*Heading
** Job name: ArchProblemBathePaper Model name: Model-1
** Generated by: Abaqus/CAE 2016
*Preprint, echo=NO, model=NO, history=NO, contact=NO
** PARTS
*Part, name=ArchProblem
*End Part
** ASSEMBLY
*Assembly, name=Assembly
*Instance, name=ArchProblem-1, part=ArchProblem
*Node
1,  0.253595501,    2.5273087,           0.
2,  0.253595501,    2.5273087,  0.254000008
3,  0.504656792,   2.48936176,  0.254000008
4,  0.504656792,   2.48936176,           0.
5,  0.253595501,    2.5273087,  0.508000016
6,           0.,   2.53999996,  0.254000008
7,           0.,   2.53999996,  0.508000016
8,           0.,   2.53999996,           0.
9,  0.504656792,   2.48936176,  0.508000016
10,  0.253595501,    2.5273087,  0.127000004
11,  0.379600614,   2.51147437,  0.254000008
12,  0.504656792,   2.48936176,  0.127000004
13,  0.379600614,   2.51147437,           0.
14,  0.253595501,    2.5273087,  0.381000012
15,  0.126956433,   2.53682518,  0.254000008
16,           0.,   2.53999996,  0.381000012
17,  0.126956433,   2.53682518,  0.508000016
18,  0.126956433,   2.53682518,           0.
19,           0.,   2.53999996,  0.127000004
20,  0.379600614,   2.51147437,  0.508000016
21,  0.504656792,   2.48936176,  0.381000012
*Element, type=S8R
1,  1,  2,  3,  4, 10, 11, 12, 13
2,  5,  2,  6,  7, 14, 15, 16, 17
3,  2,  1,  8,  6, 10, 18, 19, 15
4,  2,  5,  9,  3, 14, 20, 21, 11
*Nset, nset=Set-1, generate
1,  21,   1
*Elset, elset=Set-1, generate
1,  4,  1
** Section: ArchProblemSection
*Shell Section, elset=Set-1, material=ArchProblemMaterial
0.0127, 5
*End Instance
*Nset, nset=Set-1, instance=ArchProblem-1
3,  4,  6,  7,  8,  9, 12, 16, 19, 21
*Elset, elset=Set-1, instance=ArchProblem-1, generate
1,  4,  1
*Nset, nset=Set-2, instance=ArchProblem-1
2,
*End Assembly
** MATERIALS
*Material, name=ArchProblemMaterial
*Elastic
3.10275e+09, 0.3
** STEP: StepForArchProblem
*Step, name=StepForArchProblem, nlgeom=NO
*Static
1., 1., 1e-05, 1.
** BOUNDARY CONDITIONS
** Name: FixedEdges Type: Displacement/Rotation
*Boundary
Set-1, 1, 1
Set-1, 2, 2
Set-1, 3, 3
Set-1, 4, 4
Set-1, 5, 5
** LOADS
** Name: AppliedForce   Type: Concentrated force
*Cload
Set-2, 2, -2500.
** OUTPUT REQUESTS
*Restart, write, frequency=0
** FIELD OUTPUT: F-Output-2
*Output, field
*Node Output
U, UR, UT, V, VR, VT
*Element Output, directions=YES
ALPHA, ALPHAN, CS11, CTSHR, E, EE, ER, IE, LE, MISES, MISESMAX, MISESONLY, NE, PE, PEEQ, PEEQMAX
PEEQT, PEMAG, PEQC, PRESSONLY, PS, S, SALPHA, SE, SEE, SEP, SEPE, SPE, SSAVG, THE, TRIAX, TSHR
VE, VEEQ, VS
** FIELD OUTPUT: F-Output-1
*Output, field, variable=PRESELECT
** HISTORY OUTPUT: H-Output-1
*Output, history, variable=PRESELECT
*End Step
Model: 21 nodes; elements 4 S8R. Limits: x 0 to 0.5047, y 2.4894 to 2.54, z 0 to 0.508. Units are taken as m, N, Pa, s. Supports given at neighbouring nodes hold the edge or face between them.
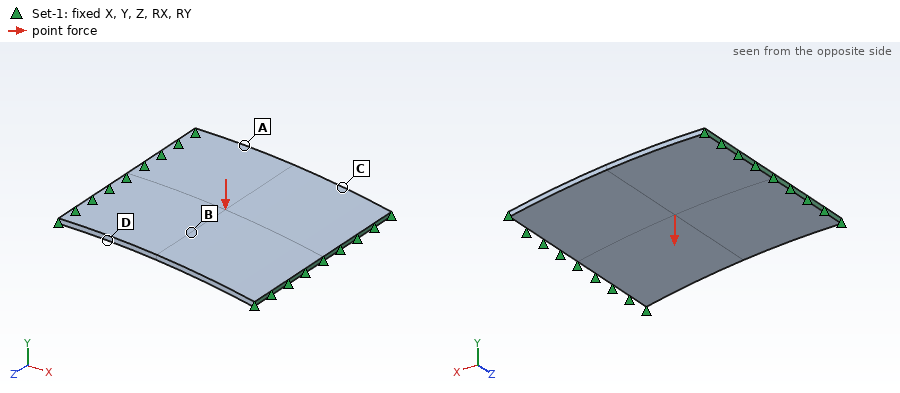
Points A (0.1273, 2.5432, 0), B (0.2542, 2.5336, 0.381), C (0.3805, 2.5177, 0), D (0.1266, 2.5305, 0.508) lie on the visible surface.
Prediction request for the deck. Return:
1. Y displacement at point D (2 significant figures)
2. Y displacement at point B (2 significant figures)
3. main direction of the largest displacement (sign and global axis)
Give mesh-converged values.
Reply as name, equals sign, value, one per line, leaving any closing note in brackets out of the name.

Y displacement at point D = -7.8e-04 m
Y displacement at point B = -0.0031 m
main direction of the largest displacement = -Y
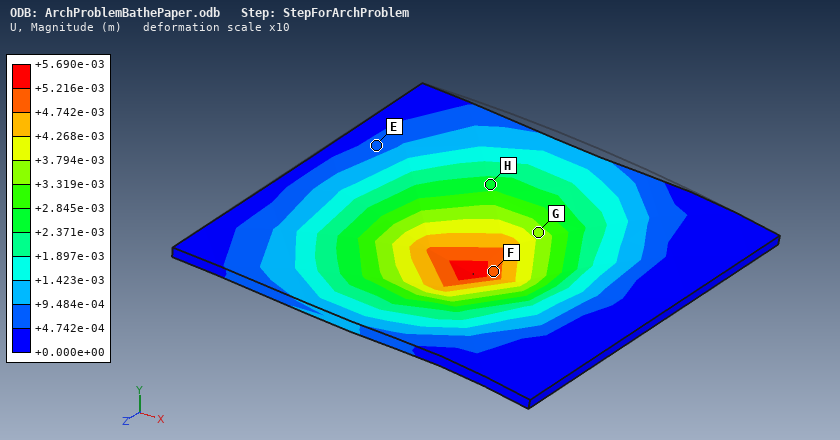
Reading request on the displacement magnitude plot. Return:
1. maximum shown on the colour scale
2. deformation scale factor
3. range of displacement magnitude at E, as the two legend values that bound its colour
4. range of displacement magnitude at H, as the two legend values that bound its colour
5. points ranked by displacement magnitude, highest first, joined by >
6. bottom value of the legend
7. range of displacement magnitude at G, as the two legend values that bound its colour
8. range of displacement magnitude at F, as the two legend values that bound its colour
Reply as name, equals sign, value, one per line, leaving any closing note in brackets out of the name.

maximum shown on the colour scale = +5.690e-03 m
deformation scale factor = 10
range of displacement magnitude at E, as the two legend values that bound its colour = +4.742e-04 to +9.484e-04 m
range of displacement magnitude at H, as the two legend values that bound its colour = +2.371e-03 to +2.845e-03 m
points ranked by displacement magnitude, highest first, joined by > = F > G > H > E
bottom value of the legend = +0.000e+00 m
range of displacement magnitude at G, as the two legend values that bound its colour = +3.319e-03 to +3.794e-03 m
range of displacement magnitude at F, as the two legend values that bound its colour = +4.742e-03 to +5.216e-03 m
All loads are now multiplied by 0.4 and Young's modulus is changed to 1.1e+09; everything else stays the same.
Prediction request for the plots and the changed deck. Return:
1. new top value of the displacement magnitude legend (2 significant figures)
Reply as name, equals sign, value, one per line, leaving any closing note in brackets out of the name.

new top value of the displacement magnitude legend = 0.0064 m
